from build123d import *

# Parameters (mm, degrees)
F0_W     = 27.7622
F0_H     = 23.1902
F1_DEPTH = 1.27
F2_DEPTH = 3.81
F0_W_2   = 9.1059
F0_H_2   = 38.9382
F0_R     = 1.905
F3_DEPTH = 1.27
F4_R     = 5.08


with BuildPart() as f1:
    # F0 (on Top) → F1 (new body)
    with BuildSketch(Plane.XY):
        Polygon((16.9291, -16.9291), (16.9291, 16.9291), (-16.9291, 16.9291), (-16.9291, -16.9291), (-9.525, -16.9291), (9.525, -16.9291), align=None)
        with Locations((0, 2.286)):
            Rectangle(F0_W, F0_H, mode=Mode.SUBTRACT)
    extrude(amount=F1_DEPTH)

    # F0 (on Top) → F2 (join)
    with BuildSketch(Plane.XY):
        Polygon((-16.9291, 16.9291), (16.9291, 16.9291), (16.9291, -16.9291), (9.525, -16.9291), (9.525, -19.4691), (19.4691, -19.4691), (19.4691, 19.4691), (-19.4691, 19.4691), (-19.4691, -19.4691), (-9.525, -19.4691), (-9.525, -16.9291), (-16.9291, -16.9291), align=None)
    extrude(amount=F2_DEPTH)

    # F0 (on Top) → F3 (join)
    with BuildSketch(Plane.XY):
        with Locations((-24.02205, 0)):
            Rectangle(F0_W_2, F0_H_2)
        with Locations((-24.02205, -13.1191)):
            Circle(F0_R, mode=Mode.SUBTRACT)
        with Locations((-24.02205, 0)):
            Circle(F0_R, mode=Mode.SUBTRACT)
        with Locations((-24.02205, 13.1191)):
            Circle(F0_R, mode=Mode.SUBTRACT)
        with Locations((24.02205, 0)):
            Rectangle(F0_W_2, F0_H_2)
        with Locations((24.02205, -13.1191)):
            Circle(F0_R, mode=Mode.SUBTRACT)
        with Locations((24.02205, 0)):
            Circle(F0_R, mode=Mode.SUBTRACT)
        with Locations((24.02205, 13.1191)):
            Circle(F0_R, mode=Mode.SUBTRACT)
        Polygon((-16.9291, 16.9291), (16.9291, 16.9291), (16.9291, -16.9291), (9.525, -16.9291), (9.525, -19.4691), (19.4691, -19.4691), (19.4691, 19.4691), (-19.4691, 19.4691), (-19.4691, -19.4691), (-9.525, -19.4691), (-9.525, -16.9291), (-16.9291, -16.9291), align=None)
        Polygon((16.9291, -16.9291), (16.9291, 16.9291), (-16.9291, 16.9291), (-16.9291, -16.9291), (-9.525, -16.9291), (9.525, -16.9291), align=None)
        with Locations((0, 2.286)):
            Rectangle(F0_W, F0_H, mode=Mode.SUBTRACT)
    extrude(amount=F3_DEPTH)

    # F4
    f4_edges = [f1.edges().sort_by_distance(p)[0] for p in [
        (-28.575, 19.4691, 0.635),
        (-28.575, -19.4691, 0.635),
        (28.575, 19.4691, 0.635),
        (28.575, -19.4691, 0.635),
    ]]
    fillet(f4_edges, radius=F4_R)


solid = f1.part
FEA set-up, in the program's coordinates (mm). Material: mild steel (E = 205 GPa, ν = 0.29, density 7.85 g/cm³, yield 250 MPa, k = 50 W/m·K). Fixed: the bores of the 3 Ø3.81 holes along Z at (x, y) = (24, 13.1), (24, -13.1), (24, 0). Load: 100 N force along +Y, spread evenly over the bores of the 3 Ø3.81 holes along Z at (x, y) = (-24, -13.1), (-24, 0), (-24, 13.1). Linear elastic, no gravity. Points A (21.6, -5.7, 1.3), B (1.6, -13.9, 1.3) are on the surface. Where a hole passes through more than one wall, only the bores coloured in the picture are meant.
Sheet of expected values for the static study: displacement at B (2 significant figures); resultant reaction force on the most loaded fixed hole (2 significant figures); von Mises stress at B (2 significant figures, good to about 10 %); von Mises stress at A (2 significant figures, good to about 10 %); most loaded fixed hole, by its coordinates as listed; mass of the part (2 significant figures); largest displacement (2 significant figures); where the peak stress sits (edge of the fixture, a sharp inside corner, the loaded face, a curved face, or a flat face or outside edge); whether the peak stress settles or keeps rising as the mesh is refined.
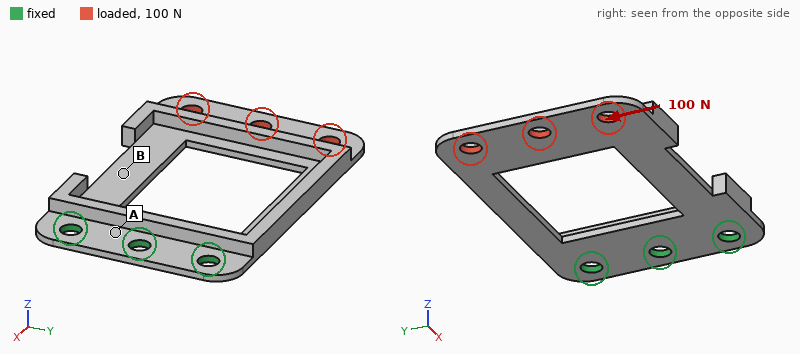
11 µm
170 N
24 MPa
11 MPa
(24, -13.1)
21 g
36 µm
a sharp inside corner
keeps rising
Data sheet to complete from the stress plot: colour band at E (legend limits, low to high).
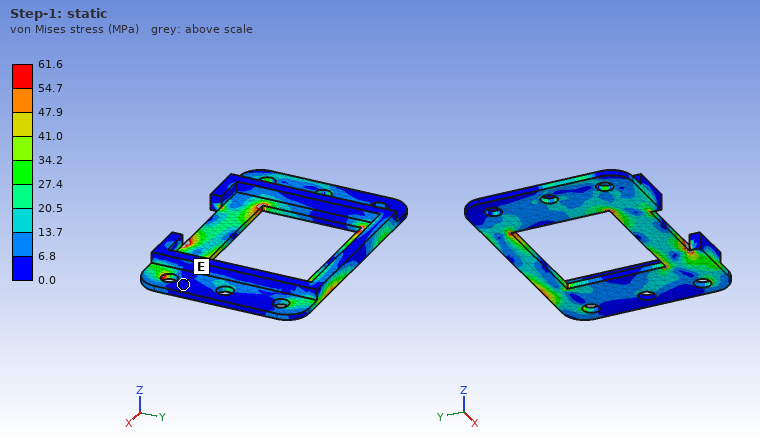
0.0 to 6.8 MPa
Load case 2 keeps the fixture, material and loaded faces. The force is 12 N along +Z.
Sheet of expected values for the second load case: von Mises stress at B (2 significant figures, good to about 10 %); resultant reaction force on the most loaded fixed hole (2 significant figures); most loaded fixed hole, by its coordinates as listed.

34 MPa
15 N
(24, 0)
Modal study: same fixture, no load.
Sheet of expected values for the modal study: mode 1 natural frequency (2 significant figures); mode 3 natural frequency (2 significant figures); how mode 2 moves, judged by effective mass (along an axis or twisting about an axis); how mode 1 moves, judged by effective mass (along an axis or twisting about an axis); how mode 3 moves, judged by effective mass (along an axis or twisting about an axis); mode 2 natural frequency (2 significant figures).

460 Hz
3200 Hz
twisting about X
along Z
along Y
1200 Hz
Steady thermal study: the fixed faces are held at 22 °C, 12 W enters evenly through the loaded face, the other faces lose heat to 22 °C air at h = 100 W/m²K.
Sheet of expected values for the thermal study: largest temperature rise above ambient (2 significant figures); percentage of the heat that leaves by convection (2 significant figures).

84 K
93 %
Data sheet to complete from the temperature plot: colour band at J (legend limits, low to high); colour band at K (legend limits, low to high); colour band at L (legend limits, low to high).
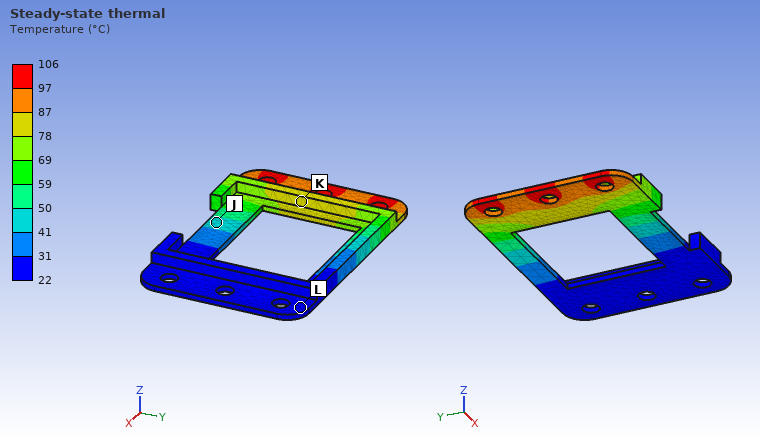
41 to 50 °C
78 to 87 °C
22 to 31 °C
